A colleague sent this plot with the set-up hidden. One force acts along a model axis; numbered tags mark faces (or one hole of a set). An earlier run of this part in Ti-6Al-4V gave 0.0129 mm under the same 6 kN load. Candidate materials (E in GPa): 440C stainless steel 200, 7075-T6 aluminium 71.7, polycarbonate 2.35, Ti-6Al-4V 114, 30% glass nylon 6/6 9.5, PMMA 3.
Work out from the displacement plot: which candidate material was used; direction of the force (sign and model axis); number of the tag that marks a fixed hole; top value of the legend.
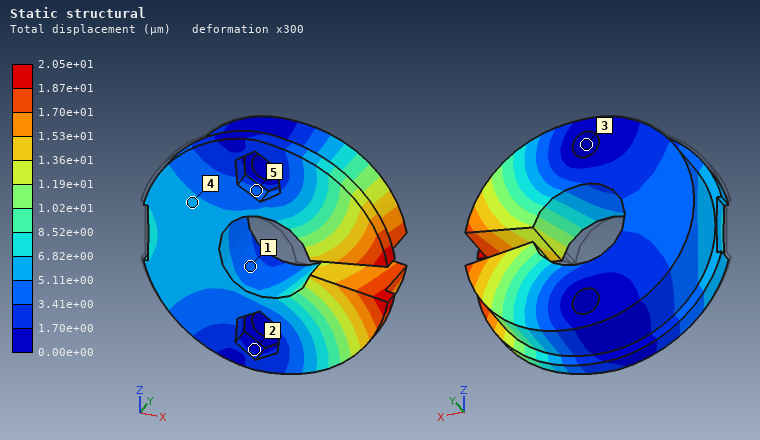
7075-T6 aluminium
+X
3
2.05e+01 µm
